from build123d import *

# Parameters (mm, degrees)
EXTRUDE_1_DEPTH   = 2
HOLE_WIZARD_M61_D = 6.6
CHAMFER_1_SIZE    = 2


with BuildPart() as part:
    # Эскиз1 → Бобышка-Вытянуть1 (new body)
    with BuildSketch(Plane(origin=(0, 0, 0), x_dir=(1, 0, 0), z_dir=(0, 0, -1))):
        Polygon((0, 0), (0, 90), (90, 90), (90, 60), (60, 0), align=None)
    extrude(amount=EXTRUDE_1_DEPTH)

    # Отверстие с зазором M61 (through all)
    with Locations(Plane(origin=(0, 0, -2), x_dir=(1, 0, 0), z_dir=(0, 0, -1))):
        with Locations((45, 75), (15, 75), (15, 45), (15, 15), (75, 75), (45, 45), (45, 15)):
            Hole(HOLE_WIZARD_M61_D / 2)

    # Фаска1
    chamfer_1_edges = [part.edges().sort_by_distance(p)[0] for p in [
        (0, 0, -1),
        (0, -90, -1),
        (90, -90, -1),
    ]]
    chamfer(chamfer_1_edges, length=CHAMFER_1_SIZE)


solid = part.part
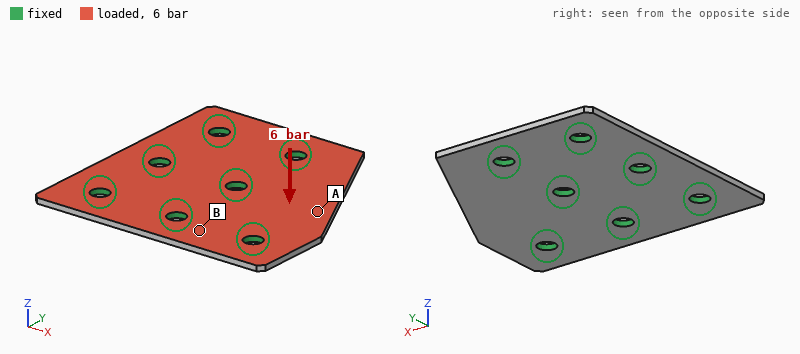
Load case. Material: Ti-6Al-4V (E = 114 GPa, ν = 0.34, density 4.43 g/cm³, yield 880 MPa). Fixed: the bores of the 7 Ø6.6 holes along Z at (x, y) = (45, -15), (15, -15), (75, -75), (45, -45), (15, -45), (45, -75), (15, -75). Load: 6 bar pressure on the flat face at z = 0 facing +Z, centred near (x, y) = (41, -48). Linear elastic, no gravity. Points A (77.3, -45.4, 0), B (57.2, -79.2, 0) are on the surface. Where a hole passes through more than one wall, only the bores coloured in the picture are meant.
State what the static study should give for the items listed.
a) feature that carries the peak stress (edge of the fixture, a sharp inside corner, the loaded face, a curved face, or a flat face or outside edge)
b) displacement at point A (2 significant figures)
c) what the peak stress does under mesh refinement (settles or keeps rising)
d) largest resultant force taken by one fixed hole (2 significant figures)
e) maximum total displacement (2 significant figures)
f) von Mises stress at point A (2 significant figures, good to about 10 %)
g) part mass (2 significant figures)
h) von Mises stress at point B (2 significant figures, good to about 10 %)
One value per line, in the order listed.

edge of the fixture
0.33 mm
keeps rising
750 N
0.42 mm
84 MPa
62 g
36 MPa
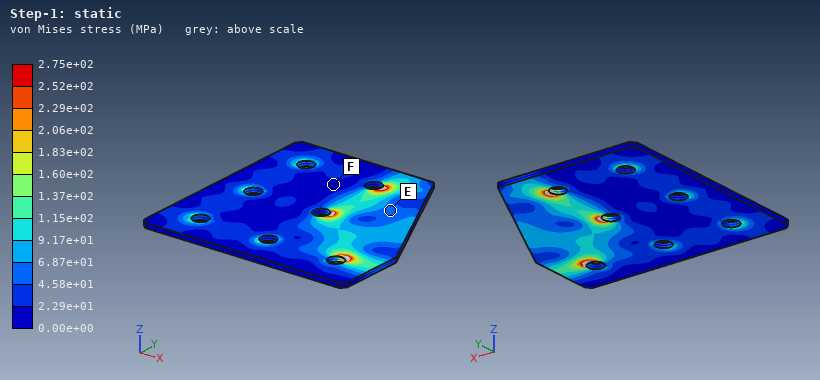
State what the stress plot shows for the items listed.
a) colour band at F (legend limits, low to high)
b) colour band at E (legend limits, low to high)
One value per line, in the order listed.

0.00e+00 to 2.29e+01 MPa
4.58e+01 to 6.87e+01 MPa
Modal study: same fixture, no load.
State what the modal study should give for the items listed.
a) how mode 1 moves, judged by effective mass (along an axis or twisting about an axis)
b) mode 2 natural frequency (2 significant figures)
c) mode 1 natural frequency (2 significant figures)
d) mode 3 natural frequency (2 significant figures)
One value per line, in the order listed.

along Z
5200 Hz
2700 Hz
7000 Hz
